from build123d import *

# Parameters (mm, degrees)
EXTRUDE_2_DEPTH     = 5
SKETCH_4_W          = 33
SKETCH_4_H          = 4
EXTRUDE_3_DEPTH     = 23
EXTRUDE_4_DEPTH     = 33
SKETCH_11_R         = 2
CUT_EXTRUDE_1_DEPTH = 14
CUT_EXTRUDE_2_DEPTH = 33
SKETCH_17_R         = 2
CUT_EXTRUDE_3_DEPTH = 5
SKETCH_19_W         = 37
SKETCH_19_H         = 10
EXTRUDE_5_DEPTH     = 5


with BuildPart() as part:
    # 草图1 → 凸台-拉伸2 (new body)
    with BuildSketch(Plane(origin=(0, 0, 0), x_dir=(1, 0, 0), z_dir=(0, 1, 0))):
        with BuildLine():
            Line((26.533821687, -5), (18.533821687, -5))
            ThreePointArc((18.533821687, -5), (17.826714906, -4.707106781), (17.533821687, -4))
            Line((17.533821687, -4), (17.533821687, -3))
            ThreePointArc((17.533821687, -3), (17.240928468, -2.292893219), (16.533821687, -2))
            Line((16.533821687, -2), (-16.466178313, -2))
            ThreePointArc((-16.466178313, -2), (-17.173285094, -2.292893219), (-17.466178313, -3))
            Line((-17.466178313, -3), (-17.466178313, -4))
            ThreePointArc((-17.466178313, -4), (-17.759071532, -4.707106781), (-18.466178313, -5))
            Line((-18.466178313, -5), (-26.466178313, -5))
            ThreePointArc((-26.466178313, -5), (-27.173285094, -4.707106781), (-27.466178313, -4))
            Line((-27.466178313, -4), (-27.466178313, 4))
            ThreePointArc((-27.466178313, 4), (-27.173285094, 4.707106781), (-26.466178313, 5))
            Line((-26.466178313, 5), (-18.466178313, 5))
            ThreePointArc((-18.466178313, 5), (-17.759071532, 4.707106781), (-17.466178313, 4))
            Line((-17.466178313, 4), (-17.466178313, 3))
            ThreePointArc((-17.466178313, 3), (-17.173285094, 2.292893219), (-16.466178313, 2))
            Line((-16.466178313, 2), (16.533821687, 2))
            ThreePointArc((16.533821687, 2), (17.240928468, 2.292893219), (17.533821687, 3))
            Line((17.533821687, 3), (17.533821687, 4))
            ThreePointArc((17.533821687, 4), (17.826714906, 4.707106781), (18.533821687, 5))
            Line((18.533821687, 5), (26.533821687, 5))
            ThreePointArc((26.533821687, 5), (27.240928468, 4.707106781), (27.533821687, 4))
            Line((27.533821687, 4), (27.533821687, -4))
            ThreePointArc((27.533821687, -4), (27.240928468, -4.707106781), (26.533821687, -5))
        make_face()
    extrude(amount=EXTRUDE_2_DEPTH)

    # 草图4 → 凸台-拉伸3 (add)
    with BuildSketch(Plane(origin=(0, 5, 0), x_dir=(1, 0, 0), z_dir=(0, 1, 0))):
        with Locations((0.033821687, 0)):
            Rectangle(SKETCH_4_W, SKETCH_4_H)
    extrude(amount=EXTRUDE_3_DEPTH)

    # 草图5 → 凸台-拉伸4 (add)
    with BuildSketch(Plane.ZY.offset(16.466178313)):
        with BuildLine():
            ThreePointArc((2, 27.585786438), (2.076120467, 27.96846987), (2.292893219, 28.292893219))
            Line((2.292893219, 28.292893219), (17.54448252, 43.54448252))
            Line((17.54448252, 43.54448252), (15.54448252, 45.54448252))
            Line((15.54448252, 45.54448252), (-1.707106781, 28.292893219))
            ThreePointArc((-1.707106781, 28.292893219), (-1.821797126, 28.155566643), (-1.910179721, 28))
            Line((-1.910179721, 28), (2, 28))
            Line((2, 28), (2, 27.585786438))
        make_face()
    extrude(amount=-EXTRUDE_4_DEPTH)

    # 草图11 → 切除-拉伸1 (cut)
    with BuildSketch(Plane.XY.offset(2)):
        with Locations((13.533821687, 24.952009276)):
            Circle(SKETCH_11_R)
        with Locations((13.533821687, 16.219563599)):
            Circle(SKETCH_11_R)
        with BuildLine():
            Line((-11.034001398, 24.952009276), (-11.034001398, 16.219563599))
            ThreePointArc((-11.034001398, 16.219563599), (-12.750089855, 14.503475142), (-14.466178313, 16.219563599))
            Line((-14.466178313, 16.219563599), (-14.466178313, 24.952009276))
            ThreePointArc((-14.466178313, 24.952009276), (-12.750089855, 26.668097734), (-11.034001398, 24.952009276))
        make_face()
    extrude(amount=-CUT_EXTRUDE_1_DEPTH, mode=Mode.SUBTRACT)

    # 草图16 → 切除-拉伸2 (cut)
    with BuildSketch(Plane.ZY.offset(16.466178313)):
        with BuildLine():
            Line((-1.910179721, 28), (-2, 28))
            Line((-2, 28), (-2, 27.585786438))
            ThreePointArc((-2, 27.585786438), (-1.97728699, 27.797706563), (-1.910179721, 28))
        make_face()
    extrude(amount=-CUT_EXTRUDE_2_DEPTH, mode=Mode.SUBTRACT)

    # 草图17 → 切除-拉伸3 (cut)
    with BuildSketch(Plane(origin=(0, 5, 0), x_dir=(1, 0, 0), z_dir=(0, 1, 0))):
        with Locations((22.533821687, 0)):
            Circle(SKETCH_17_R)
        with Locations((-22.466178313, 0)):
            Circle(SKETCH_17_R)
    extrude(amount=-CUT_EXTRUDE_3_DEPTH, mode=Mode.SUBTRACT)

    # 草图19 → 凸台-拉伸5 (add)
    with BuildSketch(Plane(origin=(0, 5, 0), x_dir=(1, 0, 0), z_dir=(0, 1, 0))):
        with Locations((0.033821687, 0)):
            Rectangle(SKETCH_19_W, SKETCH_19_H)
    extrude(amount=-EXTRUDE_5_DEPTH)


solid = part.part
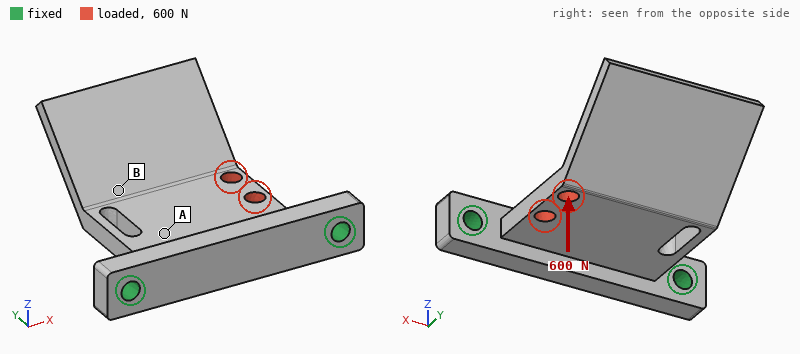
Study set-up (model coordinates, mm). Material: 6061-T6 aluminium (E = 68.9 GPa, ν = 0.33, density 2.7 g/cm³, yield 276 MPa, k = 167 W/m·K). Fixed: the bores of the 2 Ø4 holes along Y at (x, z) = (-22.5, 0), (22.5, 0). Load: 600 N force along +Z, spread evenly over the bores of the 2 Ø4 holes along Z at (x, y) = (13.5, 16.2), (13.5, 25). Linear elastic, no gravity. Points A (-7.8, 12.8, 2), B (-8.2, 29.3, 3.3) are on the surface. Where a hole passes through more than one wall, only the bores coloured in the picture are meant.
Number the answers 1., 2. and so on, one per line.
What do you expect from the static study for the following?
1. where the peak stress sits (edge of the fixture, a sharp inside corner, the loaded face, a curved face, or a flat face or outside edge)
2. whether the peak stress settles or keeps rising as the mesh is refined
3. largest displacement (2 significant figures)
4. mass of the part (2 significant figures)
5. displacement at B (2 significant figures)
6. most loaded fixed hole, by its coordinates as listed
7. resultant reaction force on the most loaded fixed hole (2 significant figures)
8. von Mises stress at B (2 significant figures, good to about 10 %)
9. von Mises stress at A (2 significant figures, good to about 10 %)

1. edge of the fixture
2. keeps rising
3. 0.66 mm
4. 20 g
5. 0.25 mm
6. (22.5, 0)
7. 520 N
8. 18 MPa
9. 63 MPa
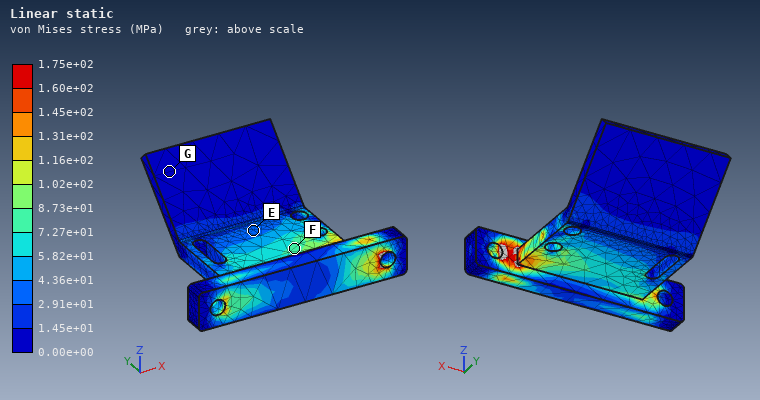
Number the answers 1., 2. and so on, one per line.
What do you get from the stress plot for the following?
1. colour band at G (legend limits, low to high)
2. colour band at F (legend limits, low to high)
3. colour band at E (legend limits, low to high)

1. 0.00e+00 to 1.45e+01 MPa
2. 7.27e+01 to 8.73e+01 MPa
3. 2.91e+01 to 4.36e+01 MPa
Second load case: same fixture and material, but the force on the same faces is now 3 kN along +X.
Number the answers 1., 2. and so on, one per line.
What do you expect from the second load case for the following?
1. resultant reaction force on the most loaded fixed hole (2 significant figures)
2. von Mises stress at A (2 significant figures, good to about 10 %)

1. 2.1 kN
2. 41 MPa
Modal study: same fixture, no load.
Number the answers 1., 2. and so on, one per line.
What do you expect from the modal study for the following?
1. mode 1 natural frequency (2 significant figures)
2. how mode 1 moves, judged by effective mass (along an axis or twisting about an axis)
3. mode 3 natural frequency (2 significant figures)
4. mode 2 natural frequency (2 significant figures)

1. 1400 Hz
2. along Z
3. 5300 Hz
4. 3700 Hz
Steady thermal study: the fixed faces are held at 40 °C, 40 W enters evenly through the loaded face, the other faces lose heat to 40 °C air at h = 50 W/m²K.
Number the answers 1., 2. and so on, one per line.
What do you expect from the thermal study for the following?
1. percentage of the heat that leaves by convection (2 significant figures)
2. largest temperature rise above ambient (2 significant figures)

1. 19 %
2. 70 K
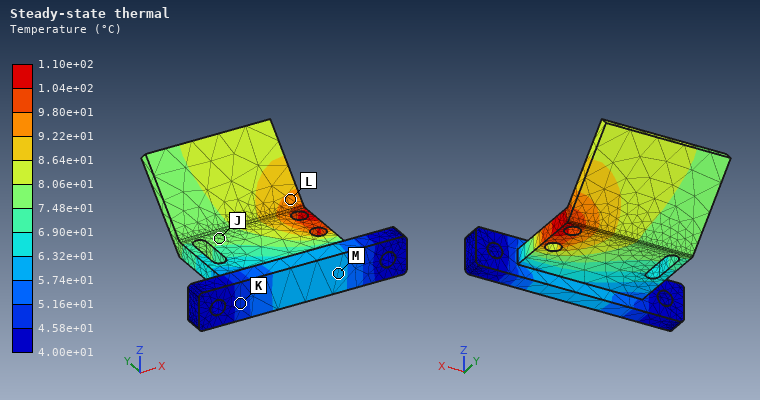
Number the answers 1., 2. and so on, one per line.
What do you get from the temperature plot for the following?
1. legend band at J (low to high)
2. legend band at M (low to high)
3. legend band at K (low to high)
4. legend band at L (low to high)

1. 7.48e+01 to 8.06e+01 °C
2. 5.74e+01 to 6.32e+01 °C
3. 4.58e+01 to 5.16e+01 °C
4. 9.22e+01 to 9.80e+01 °C
